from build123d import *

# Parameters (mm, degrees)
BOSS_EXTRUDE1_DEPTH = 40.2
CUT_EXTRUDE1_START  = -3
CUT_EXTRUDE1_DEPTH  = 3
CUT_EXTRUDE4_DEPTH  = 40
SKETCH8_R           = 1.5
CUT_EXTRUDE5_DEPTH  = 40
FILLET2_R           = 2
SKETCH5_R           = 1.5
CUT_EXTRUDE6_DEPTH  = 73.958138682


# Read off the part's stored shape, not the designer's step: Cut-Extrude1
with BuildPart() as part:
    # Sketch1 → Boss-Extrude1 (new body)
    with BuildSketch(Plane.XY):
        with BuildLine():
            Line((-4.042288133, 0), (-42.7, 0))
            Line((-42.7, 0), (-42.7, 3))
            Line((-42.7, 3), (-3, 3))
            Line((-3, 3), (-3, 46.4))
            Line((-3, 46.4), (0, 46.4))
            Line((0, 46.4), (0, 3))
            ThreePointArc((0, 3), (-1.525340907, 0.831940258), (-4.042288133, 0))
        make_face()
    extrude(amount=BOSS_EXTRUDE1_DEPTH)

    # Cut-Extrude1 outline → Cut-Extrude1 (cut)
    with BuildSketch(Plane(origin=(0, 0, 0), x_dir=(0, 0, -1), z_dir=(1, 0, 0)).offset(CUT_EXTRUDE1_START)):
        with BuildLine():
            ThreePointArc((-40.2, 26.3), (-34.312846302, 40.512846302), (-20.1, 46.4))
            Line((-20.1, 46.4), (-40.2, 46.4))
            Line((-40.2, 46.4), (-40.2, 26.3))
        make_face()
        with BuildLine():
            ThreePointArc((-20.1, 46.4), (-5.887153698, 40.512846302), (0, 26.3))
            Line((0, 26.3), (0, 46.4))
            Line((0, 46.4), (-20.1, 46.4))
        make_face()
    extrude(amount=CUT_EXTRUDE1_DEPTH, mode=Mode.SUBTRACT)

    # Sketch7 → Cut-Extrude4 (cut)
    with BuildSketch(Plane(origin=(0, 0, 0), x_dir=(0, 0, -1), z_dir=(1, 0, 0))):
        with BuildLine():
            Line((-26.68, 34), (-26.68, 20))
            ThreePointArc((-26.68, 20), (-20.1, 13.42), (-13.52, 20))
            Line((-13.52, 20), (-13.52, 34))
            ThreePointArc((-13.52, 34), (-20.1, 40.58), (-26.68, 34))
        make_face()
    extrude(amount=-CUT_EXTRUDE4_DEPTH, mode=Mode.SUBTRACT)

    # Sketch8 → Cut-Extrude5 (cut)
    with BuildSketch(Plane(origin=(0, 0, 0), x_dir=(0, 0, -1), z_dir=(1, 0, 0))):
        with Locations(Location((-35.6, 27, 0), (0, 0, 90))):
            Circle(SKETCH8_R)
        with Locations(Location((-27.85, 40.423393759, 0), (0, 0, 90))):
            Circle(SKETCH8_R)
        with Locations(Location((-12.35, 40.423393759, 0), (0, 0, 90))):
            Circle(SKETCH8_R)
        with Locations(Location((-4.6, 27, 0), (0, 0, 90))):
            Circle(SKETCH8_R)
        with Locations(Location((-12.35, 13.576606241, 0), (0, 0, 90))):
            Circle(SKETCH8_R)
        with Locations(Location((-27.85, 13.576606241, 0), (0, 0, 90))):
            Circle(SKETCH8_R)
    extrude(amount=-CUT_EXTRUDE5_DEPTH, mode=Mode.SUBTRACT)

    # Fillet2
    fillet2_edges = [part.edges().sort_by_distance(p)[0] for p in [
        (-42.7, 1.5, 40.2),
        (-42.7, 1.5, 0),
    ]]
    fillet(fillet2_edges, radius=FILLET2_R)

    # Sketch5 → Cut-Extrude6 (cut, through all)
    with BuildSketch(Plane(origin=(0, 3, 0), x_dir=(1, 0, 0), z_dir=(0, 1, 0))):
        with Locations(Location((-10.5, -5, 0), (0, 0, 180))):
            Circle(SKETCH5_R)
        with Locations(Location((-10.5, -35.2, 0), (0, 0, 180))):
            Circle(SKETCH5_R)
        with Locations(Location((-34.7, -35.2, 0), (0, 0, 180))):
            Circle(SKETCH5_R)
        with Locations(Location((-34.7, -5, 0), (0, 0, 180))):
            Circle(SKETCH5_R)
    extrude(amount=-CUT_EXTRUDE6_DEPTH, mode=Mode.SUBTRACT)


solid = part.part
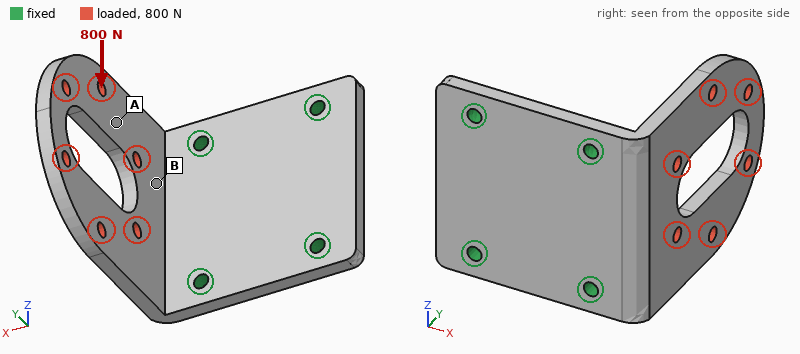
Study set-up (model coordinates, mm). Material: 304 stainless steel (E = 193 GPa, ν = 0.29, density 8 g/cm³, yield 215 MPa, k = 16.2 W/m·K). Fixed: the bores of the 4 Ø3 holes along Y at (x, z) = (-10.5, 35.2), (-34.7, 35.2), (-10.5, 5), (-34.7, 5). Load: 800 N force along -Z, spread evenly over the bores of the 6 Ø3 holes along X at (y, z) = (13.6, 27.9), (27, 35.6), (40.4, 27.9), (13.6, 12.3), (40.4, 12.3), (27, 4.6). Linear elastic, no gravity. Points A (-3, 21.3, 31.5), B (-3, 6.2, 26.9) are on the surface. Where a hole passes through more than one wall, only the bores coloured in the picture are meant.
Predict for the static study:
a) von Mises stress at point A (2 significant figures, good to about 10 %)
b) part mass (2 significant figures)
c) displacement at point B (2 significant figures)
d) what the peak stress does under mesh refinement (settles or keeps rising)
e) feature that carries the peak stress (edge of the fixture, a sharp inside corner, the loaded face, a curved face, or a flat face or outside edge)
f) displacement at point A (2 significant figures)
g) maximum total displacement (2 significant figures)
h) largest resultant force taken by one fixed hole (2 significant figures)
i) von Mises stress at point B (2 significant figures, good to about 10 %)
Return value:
27 MPa
68 g
10 µm
keeps rising
edge of the fixture
36 µm
68 µm
800 N
56 MPa
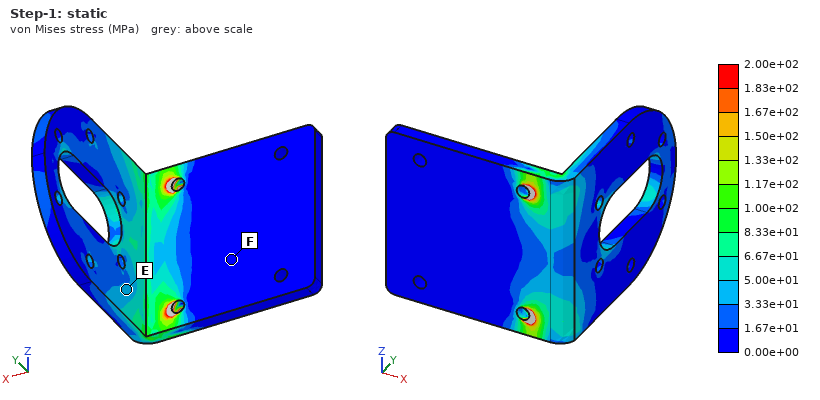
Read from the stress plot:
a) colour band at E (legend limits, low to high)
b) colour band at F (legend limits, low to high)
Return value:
3.33e+01 to 5.00e+01 MPa
0.00e+00 to 1.67e+01 MPa
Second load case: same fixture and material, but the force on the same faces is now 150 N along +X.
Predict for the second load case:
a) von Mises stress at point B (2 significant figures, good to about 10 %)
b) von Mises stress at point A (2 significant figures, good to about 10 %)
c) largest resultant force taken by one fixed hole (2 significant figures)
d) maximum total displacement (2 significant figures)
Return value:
47 MPa
32 MPa
55 N
0.22 mm
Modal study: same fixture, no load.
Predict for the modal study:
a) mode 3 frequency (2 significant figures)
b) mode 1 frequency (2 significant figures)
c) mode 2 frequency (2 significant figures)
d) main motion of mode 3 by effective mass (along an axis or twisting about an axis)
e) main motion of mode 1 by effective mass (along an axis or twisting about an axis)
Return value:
4700 Hz
1100 Hz
3000 Hz
along Z
along X
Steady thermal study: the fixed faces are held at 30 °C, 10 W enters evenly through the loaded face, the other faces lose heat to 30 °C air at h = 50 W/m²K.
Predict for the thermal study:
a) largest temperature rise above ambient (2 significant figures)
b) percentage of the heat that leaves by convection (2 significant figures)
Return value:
77 K
76 %
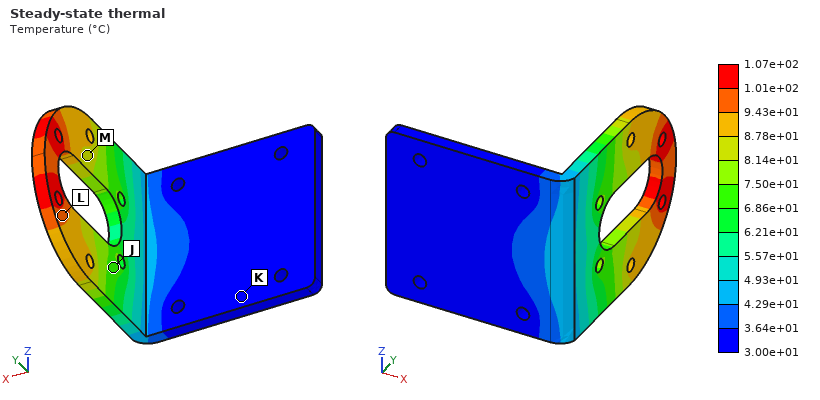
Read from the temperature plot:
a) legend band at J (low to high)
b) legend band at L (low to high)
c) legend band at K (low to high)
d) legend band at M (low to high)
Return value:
6.86e+01 to 7.50e+01 °C
9.43e+01 to 1.01e+02 °C
3.00e+01 to 3.64e+01 °C
8.14e+01 to 8.78e+01 °C
